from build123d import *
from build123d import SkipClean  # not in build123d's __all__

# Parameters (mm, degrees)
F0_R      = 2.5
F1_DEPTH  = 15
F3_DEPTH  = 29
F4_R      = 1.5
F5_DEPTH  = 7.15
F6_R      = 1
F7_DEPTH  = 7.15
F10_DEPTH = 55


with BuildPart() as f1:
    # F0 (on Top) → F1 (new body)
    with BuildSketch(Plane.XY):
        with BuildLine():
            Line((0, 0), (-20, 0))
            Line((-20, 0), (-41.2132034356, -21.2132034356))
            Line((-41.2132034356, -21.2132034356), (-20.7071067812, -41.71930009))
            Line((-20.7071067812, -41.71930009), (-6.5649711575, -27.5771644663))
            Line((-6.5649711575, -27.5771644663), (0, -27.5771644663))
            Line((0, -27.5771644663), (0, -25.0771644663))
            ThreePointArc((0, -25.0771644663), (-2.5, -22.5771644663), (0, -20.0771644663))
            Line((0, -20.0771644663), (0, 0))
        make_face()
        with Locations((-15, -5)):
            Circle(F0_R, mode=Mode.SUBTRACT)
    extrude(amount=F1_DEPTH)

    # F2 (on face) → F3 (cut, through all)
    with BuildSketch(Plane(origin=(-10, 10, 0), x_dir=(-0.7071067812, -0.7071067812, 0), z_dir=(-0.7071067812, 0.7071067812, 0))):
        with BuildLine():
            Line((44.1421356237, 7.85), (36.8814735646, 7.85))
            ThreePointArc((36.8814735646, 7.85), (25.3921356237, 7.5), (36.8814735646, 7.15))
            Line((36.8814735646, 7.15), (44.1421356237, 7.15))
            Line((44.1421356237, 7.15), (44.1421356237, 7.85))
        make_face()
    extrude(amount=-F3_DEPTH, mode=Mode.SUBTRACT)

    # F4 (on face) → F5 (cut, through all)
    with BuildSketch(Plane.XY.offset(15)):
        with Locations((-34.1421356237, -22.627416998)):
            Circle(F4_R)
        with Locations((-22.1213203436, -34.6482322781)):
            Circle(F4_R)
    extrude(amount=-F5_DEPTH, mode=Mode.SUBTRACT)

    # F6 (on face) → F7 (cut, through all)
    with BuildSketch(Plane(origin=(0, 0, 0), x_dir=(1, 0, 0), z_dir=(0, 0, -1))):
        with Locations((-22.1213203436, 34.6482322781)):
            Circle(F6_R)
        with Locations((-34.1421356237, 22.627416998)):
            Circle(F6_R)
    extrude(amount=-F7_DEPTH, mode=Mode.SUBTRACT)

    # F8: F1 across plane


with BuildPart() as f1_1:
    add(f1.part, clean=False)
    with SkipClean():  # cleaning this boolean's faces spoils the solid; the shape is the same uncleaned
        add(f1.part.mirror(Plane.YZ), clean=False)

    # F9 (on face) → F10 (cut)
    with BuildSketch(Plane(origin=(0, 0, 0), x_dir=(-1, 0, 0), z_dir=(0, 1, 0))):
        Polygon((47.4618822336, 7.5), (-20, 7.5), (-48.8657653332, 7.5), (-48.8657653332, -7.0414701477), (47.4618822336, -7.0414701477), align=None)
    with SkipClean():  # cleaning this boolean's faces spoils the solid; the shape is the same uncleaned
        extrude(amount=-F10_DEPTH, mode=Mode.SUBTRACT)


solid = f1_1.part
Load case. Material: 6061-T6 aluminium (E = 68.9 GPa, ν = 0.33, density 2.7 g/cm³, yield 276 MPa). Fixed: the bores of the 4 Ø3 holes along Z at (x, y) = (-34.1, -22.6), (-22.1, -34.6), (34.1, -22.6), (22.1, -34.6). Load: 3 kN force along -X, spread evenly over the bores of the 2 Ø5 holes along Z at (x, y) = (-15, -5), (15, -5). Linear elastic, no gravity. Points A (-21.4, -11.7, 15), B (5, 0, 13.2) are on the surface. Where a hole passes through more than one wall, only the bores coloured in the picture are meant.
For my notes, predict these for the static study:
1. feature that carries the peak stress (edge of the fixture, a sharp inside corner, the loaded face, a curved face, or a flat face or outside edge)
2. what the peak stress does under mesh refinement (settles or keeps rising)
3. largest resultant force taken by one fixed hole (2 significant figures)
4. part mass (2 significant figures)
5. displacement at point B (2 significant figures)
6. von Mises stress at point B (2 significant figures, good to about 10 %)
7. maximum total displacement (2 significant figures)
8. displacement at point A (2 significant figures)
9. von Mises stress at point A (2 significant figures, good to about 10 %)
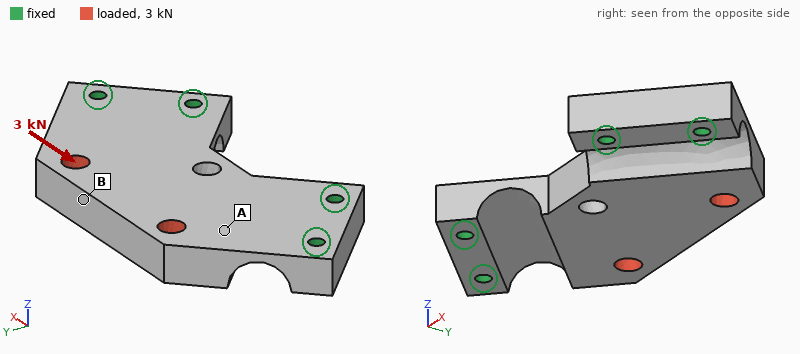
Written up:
edge of the fixture
keeps rising
1.3 kN
34 g
16 µm
8.0 MPa
19 µm
11 µm
24 MPa
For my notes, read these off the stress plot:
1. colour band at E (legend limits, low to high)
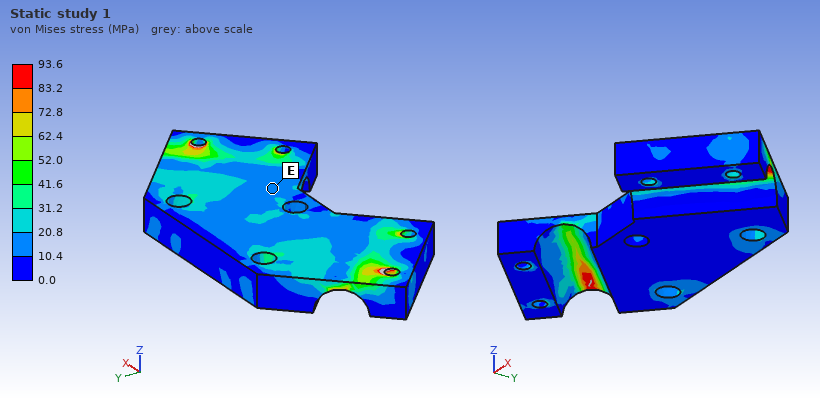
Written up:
10.4 to 20.8 MPa
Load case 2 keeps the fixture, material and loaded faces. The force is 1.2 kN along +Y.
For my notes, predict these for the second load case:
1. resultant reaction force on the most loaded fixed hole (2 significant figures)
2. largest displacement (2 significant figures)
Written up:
520 N
63 µm
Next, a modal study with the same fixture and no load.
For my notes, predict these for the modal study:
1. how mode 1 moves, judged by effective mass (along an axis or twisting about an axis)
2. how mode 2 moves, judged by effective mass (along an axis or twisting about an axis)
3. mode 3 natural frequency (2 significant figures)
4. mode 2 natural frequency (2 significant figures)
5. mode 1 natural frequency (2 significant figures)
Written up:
along Z
twisting about Y
11 kHz
9400 Hz
2700 Hz
